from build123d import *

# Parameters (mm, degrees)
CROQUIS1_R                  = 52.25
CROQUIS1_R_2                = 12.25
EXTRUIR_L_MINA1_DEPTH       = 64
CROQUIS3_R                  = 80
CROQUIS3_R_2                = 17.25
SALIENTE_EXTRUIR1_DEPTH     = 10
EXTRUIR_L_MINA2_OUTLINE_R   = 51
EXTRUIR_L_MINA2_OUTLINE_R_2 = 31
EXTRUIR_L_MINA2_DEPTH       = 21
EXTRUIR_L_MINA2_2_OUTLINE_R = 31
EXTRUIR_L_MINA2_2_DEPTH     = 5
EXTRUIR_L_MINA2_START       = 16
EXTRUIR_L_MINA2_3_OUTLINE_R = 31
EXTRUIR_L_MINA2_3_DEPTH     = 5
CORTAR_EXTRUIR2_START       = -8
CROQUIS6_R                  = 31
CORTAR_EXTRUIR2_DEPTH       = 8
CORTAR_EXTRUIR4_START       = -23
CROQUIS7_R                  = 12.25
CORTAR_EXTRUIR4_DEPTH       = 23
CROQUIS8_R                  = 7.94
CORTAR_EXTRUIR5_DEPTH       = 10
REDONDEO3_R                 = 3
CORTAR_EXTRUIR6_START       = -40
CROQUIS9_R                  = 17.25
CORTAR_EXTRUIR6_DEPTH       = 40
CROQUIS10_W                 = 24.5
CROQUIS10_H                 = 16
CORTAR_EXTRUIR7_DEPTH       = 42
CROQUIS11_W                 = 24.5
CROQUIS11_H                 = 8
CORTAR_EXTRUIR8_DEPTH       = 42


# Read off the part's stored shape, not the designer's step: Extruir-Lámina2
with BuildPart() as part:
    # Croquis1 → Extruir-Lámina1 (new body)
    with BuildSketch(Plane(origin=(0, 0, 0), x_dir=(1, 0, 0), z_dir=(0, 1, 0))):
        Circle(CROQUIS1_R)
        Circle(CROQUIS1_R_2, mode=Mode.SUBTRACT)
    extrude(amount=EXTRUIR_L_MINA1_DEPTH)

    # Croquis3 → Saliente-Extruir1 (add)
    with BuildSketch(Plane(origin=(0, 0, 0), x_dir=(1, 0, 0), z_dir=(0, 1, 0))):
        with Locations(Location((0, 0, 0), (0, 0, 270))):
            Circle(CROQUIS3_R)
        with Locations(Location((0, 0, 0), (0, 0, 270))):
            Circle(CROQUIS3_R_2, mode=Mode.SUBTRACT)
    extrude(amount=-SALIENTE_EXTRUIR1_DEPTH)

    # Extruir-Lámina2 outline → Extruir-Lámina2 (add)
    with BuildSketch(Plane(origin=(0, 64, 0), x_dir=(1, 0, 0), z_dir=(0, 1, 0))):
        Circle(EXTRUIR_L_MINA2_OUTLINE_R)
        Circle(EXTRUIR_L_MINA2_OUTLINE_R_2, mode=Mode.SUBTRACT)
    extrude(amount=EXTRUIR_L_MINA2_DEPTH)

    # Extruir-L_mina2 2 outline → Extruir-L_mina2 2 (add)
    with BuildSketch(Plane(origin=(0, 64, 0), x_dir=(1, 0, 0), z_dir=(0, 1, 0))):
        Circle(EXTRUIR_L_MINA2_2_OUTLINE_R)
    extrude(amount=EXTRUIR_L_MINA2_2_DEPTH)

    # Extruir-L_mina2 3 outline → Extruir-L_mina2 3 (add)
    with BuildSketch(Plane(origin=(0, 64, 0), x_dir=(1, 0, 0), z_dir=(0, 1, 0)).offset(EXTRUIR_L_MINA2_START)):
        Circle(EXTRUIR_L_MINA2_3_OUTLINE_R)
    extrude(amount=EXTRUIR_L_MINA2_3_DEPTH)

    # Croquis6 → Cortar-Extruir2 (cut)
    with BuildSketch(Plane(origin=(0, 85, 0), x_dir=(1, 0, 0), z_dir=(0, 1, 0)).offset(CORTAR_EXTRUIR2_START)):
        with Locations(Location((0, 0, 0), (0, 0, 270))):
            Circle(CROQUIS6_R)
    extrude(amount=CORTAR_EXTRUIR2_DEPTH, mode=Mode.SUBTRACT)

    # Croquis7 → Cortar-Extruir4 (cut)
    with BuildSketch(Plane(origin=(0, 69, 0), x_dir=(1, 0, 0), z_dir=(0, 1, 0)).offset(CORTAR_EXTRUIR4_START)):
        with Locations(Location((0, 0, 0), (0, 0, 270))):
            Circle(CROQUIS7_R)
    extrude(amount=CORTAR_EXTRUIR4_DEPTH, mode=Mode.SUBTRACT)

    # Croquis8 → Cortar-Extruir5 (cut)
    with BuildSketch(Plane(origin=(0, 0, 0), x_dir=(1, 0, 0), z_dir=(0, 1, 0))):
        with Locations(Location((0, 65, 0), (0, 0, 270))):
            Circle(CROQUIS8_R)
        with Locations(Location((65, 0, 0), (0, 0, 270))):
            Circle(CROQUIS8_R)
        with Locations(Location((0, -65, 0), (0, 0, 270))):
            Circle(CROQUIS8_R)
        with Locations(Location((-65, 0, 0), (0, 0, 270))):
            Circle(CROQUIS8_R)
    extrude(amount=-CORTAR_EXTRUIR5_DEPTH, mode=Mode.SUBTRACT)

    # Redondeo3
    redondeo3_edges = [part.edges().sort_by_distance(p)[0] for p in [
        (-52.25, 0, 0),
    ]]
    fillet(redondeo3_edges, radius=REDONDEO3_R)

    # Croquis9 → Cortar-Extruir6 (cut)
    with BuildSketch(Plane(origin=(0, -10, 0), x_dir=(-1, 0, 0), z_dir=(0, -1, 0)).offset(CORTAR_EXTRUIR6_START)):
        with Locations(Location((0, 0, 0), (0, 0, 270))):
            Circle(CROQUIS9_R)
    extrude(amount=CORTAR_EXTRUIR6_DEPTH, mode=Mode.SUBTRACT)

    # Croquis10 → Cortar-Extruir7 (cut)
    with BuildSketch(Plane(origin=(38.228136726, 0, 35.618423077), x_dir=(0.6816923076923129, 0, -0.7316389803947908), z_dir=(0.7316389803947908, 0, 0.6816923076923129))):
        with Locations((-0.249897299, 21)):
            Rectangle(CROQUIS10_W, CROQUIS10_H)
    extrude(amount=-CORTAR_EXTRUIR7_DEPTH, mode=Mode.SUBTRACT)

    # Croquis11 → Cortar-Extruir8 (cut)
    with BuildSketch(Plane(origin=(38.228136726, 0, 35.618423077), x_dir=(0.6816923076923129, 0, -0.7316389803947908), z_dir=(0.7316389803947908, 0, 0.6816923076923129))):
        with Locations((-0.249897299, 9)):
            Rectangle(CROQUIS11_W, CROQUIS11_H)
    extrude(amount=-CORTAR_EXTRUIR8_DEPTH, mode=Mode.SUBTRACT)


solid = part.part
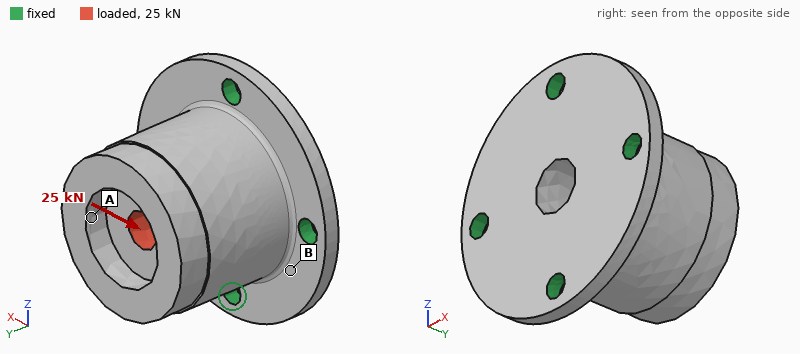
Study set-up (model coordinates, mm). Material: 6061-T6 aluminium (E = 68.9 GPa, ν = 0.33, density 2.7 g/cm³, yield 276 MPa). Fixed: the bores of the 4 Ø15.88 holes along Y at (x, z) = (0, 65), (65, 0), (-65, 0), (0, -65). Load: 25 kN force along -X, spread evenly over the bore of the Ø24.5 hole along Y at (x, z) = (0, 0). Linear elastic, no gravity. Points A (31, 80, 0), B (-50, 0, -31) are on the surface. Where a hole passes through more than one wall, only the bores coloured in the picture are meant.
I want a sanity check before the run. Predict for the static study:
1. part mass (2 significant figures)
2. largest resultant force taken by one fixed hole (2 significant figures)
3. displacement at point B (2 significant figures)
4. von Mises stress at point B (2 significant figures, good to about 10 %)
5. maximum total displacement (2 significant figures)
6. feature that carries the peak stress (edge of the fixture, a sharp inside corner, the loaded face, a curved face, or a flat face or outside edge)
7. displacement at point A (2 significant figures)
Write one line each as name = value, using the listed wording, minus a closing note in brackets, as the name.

part mass = 2.1 kg
largest resultant force taken by one fixed hole = 15 kN
displacement at point B = 21 µm
von Mises stress at point B = 16 MPa
maximum total displacement = 66 µm
feature that carries the peak stress = a curved face
displacement at point A = 58 µm
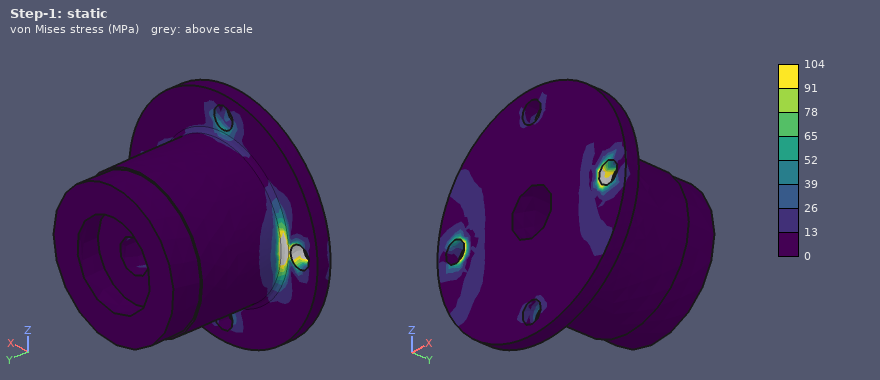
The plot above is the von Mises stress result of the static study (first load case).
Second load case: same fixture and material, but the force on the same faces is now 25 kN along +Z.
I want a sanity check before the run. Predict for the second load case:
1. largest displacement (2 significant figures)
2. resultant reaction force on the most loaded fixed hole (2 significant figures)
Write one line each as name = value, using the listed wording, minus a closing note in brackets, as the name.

largest displacement = 65 µm
resultant reaction force on the most loaded fixed hole = 15 kN
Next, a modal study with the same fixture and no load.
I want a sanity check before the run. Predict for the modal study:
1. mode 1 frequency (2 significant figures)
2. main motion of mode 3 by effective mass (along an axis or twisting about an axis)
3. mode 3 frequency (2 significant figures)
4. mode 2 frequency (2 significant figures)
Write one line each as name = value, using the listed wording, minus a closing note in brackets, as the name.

mode 1 frequency = 3000 Hz
main motion of mode 3 by effective mass = along Y
mode 3 frequency = 4400 Hz
mode 2 frequency = 3100 Hz
